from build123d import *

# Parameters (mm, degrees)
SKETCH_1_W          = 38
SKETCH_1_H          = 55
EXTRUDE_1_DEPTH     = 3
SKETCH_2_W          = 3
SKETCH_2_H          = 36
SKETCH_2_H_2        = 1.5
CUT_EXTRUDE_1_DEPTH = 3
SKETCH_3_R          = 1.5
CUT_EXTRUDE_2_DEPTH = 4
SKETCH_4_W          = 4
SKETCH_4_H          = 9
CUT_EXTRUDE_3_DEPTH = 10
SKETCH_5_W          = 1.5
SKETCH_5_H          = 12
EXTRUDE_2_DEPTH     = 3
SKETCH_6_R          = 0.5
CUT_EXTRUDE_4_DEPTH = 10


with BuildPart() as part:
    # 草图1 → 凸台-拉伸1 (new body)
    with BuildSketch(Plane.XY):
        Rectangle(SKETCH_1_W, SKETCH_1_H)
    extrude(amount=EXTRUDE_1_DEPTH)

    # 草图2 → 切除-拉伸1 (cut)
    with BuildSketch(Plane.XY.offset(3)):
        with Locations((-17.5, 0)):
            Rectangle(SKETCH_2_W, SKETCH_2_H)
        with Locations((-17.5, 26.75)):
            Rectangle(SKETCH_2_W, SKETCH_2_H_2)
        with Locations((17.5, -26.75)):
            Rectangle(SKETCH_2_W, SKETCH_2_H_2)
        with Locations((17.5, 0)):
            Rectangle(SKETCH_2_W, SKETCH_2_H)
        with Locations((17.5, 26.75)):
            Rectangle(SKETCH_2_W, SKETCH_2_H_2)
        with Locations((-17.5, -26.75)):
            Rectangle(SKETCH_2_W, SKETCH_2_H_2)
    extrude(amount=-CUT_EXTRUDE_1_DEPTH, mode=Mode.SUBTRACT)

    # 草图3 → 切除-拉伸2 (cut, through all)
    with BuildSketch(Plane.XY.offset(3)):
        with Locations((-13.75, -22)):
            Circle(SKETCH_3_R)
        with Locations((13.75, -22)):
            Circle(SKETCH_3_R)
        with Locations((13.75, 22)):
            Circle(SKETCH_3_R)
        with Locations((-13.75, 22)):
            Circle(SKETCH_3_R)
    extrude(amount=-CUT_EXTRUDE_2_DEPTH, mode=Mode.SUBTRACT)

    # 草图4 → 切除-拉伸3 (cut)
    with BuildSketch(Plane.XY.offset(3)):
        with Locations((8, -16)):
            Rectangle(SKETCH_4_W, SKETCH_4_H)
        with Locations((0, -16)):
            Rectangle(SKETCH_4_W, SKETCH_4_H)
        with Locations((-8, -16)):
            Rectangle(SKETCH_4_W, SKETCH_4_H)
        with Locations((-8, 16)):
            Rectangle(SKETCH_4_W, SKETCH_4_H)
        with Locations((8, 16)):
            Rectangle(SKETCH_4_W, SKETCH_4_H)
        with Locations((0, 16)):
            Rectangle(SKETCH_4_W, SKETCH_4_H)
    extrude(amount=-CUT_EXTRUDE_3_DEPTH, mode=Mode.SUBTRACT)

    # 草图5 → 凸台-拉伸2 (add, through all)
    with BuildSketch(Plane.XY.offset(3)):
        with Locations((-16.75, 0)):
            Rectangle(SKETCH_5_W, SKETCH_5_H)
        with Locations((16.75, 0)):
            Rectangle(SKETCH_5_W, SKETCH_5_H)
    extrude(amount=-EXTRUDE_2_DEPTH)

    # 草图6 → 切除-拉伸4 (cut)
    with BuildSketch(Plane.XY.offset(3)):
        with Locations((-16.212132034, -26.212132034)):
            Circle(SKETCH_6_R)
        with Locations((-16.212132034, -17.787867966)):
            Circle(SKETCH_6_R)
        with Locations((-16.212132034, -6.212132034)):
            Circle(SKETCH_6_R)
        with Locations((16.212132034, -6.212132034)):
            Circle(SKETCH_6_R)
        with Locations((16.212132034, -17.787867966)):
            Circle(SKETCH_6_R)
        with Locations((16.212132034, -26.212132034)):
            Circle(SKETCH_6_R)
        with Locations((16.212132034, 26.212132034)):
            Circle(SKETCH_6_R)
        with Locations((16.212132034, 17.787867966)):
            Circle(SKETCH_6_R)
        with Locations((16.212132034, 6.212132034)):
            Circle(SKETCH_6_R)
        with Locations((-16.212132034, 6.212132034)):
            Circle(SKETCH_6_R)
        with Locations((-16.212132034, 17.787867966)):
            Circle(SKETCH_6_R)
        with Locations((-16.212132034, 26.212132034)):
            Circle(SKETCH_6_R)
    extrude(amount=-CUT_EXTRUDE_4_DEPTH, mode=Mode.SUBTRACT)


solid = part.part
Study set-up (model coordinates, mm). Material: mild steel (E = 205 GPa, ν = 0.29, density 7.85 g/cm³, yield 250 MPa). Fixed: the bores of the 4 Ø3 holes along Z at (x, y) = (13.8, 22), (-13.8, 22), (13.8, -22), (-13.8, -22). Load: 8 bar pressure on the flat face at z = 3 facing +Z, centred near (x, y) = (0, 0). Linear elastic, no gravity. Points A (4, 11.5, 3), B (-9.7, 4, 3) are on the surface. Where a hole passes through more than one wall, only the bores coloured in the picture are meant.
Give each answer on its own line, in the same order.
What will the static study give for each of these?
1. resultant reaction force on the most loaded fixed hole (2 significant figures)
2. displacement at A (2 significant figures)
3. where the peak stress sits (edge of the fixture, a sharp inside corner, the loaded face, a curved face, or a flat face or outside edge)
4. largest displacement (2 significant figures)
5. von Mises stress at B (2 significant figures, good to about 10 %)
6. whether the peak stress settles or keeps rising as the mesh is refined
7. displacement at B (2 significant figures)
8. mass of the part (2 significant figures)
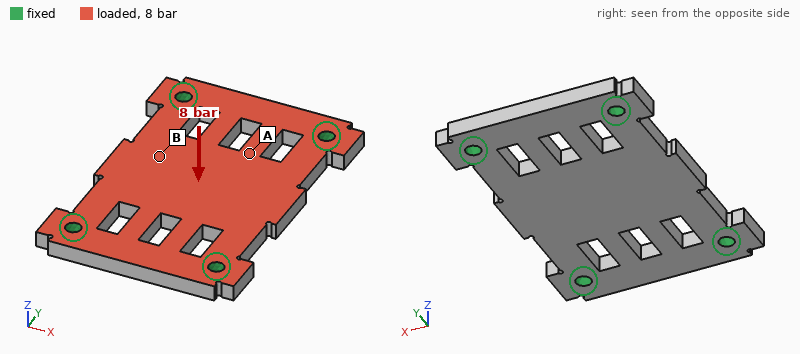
330 N
17 µm
edge of the fixture
24 µm
42 MPa
keeps rising
22 µm
39 g
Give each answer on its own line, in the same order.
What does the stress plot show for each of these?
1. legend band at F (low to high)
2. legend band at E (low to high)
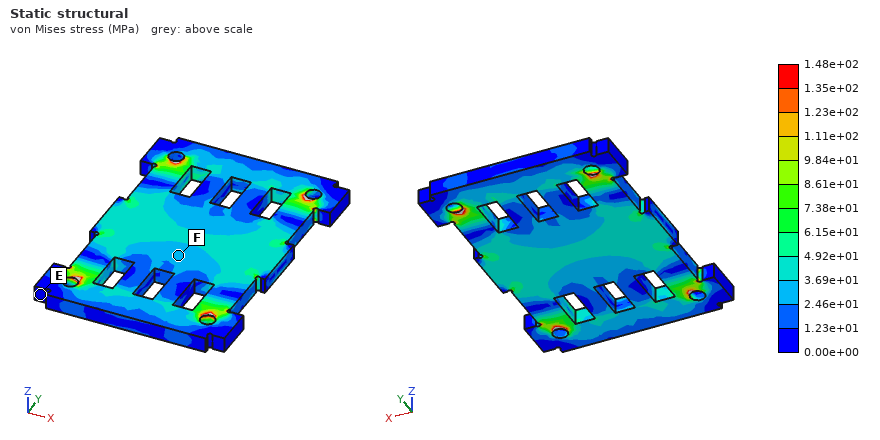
2.46e+01 to 3.69e+01 MPa
0.00e+00 to 1.23e+01 MPa
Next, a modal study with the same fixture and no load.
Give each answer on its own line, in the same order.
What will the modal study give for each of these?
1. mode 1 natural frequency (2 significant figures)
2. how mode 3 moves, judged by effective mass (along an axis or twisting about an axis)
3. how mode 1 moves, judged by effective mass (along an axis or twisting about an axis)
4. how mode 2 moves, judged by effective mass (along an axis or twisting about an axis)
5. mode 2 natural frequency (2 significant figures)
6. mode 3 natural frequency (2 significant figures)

6700 Hz
twisting about X
along Z
twisting about Y
9400 Hz
16 kHz
